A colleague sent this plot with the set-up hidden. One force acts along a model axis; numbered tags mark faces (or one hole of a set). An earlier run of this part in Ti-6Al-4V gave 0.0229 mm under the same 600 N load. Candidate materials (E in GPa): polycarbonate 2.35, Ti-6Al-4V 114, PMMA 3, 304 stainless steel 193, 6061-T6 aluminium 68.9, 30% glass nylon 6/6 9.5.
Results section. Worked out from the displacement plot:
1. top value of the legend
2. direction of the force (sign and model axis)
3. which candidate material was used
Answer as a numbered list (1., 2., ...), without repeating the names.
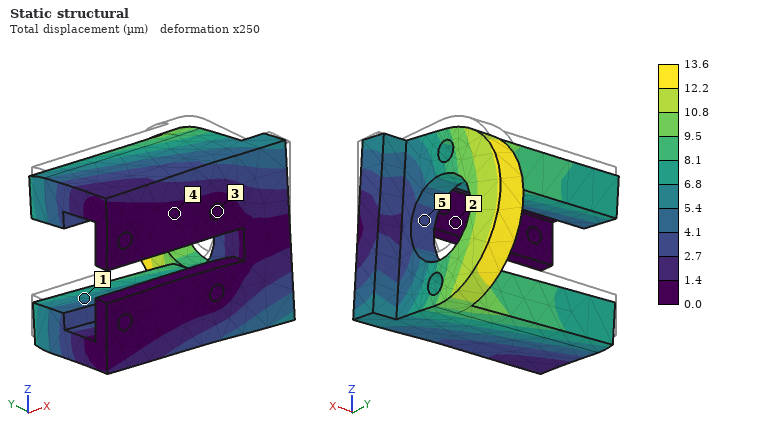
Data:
1. 13.6 µm
2. -Z
3. 304 stainless steel
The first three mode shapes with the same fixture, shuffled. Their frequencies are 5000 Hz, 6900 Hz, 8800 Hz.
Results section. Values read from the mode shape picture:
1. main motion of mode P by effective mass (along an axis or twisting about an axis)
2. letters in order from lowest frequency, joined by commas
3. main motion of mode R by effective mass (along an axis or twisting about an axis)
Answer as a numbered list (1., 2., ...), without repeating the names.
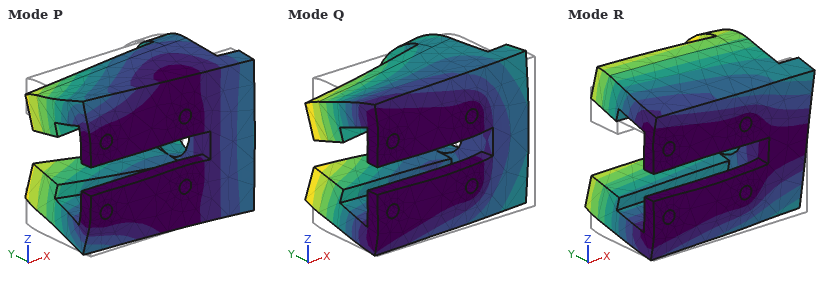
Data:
1. along X
2. R, P, Q
3. along Z
